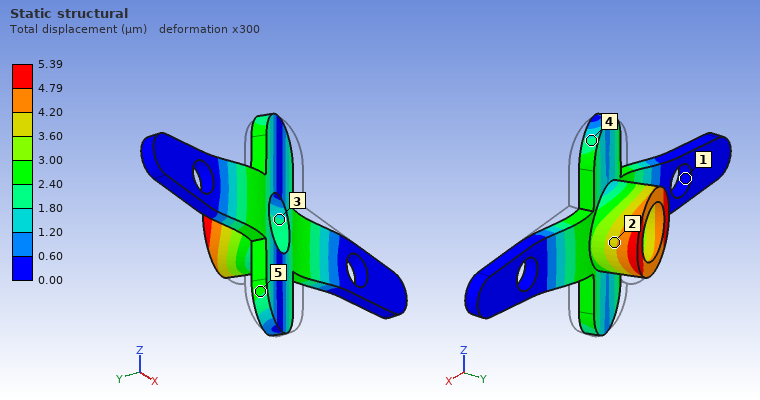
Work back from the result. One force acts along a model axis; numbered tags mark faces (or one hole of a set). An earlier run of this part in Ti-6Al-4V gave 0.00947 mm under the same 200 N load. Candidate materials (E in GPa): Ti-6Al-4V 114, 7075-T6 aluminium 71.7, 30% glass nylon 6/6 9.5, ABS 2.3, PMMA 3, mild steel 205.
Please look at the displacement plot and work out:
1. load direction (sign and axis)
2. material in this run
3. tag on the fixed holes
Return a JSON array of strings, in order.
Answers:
["-X", "mild steel", "1"]
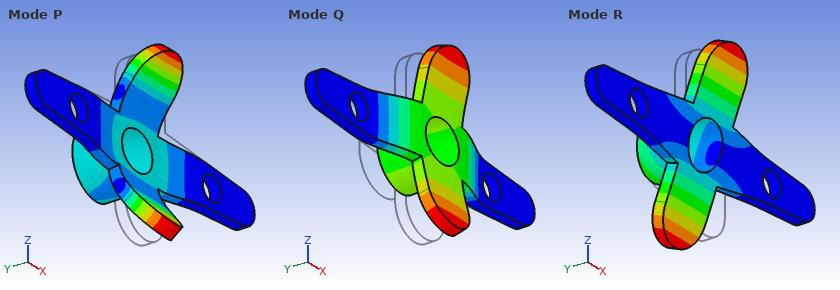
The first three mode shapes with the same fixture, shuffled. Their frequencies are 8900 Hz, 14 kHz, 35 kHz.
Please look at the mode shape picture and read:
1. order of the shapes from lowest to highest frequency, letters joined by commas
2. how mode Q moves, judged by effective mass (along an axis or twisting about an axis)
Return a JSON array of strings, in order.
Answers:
["R, Q, P", "along Y"]
